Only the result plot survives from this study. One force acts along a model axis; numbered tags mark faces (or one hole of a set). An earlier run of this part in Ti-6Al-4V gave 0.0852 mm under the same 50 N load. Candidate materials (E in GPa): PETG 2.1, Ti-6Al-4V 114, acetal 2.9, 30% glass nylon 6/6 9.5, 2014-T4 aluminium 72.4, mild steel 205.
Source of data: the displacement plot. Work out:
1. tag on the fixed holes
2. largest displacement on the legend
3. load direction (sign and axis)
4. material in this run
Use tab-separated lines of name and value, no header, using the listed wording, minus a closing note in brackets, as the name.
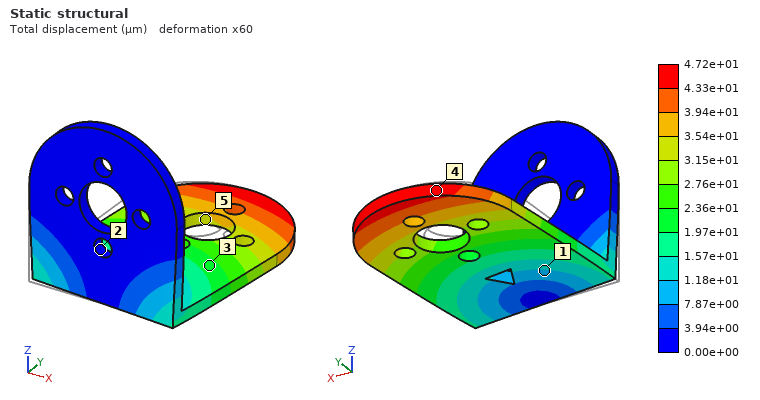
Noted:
tag on the fixed holes	2
largest displacement on the legend	4.72e+01 µm
load direction	+X
material in this run	mild steel
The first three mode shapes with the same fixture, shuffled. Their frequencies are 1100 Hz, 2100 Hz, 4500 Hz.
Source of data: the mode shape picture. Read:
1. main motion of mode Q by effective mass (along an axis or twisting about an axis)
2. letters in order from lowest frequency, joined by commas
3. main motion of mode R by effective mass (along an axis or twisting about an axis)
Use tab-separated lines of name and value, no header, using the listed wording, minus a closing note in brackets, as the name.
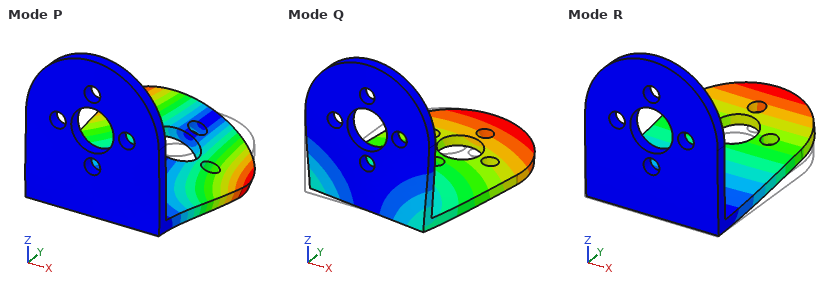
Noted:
main motion of mode Q by effective mass	along X
letters in order from lowest frequency, joined by commas	R, Q, P
main motion of mode R by effective mass	along Z
